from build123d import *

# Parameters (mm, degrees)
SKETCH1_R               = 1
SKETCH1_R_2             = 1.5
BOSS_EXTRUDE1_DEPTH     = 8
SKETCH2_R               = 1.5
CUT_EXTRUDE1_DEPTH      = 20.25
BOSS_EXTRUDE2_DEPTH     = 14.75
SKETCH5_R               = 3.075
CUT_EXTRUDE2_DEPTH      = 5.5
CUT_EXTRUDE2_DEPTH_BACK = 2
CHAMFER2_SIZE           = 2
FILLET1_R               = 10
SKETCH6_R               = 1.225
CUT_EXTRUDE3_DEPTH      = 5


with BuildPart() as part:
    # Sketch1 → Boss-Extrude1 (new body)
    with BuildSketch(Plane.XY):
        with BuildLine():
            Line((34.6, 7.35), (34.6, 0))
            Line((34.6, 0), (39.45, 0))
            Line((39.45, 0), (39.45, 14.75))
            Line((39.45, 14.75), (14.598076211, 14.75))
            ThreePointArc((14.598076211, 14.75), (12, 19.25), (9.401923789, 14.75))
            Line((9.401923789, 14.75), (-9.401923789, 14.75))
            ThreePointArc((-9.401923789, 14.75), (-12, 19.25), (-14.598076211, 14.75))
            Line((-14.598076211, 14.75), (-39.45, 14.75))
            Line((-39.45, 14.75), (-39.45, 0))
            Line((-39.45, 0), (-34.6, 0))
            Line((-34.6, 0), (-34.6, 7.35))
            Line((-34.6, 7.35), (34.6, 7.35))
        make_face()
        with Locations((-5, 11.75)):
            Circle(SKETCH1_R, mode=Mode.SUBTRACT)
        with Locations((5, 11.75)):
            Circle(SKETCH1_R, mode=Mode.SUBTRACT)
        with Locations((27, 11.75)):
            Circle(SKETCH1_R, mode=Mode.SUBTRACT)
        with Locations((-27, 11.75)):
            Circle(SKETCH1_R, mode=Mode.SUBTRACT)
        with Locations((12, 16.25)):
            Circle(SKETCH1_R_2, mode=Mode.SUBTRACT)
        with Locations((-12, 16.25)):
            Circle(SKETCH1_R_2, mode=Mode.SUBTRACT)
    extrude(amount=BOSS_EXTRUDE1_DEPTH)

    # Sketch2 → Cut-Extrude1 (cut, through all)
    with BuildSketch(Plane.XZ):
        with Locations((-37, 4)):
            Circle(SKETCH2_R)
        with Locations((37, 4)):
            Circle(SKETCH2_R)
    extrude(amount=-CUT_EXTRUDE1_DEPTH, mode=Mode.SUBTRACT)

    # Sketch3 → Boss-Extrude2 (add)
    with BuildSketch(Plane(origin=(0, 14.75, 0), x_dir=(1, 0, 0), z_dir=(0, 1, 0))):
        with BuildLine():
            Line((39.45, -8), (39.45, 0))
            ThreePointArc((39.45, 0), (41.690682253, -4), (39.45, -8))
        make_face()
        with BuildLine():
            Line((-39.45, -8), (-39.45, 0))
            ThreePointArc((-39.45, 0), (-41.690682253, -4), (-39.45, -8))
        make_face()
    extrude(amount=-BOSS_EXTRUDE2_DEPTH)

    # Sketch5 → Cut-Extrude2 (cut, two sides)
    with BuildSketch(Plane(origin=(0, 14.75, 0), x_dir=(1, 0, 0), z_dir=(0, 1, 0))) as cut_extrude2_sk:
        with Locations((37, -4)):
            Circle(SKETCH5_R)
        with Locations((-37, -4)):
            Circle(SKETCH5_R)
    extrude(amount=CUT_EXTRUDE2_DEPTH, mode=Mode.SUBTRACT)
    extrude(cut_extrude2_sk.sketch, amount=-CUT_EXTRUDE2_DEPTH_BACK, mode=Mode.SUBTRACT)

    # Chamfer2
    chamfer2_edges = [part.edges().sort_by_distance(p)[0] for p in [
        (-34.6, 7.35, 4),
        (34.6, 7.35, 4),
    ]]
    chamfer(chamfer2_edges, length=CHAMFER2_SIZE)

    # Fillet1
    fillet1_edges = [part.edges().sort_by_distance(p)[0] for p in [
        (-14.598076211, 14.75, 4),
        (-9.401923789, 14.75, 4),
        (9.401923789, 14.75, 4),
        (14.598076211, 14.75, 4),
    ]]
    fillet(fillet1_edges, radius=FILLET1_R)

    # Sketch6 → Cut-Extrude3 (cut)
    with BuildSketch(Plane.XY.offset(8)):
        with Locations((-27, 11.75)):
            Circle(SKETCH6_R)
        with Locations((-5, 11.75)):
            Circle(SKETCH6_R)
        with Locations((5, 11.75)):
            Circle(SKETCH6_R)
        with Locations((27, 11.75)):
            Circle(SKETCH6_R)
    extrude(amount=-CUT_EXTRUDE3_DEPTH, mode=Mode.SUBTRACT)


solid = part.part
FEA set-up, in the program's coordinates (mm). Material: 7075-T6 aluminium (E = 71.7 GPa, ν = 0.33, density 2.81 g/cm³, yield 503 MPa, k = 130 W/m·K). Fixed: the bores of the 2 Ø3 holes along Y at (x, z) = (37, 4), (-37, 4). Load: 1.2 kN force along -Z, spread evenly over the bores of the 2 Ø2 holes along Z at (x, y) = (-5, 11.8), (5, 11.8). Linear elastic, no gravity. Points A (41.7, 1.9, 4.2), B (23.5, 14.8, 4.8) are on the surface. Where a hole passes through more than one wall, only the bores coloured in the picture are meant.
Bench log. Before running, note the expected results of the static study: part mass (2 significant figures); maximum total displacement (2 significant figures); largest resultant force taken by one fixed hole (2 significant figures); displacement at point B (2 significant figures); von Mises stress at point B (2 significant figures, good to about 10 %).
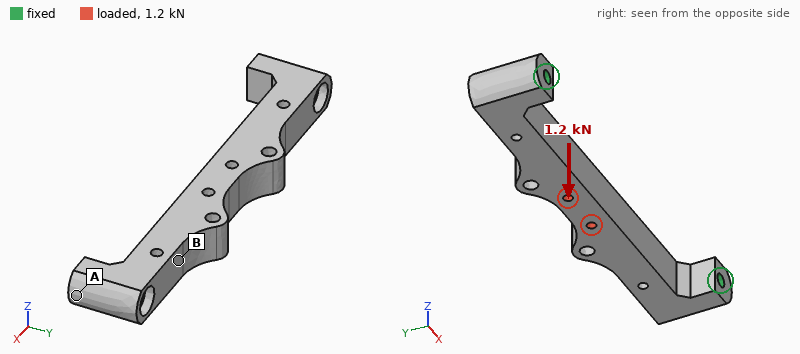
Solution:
16 g
0.15 mm
600 N
0.052 mm
42 MPa
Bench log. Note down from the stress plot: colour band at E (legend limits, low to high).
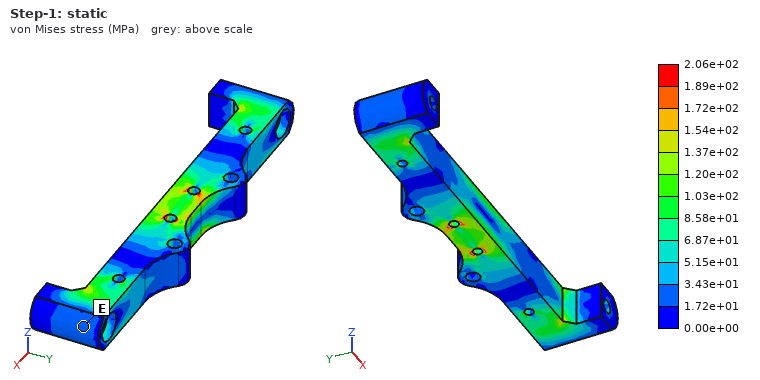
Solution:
1.72e+01 to 3.43e+01 MPa
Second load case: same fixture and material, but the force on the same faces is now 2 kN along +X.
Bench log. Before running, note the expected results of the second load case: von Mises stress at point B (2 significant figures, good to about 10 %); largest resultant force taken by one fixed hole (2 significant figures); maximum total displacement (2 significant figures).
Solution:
19 MPa
1.0 kN
13 µm
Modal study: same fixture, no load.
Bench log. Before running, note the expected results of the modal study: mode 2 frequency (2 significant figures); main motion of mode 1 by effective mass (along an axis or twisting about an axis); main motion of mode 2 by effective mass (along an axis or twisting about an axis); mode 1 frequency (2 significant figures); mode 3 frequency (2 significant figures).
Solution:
6500 Hz
along Z
along Y
6000 Hz
16 kHz
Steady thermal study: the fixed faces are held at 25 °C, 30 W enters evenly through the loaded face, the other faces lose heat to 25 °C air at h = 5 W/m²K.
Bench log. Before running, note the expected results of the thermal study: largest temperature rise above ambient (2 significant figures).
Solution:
68 K
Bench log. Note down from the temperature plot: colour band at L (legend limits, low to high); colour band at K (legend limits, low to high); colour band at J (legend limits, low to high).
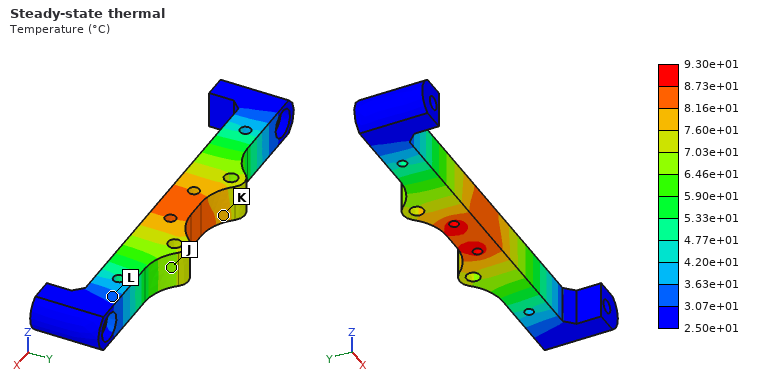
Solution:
3.07e+01 to 3.63e+01 °C
7.60e+01 to 8.16e+01 °C
6.46e+01 to 7.03e+01 °C
